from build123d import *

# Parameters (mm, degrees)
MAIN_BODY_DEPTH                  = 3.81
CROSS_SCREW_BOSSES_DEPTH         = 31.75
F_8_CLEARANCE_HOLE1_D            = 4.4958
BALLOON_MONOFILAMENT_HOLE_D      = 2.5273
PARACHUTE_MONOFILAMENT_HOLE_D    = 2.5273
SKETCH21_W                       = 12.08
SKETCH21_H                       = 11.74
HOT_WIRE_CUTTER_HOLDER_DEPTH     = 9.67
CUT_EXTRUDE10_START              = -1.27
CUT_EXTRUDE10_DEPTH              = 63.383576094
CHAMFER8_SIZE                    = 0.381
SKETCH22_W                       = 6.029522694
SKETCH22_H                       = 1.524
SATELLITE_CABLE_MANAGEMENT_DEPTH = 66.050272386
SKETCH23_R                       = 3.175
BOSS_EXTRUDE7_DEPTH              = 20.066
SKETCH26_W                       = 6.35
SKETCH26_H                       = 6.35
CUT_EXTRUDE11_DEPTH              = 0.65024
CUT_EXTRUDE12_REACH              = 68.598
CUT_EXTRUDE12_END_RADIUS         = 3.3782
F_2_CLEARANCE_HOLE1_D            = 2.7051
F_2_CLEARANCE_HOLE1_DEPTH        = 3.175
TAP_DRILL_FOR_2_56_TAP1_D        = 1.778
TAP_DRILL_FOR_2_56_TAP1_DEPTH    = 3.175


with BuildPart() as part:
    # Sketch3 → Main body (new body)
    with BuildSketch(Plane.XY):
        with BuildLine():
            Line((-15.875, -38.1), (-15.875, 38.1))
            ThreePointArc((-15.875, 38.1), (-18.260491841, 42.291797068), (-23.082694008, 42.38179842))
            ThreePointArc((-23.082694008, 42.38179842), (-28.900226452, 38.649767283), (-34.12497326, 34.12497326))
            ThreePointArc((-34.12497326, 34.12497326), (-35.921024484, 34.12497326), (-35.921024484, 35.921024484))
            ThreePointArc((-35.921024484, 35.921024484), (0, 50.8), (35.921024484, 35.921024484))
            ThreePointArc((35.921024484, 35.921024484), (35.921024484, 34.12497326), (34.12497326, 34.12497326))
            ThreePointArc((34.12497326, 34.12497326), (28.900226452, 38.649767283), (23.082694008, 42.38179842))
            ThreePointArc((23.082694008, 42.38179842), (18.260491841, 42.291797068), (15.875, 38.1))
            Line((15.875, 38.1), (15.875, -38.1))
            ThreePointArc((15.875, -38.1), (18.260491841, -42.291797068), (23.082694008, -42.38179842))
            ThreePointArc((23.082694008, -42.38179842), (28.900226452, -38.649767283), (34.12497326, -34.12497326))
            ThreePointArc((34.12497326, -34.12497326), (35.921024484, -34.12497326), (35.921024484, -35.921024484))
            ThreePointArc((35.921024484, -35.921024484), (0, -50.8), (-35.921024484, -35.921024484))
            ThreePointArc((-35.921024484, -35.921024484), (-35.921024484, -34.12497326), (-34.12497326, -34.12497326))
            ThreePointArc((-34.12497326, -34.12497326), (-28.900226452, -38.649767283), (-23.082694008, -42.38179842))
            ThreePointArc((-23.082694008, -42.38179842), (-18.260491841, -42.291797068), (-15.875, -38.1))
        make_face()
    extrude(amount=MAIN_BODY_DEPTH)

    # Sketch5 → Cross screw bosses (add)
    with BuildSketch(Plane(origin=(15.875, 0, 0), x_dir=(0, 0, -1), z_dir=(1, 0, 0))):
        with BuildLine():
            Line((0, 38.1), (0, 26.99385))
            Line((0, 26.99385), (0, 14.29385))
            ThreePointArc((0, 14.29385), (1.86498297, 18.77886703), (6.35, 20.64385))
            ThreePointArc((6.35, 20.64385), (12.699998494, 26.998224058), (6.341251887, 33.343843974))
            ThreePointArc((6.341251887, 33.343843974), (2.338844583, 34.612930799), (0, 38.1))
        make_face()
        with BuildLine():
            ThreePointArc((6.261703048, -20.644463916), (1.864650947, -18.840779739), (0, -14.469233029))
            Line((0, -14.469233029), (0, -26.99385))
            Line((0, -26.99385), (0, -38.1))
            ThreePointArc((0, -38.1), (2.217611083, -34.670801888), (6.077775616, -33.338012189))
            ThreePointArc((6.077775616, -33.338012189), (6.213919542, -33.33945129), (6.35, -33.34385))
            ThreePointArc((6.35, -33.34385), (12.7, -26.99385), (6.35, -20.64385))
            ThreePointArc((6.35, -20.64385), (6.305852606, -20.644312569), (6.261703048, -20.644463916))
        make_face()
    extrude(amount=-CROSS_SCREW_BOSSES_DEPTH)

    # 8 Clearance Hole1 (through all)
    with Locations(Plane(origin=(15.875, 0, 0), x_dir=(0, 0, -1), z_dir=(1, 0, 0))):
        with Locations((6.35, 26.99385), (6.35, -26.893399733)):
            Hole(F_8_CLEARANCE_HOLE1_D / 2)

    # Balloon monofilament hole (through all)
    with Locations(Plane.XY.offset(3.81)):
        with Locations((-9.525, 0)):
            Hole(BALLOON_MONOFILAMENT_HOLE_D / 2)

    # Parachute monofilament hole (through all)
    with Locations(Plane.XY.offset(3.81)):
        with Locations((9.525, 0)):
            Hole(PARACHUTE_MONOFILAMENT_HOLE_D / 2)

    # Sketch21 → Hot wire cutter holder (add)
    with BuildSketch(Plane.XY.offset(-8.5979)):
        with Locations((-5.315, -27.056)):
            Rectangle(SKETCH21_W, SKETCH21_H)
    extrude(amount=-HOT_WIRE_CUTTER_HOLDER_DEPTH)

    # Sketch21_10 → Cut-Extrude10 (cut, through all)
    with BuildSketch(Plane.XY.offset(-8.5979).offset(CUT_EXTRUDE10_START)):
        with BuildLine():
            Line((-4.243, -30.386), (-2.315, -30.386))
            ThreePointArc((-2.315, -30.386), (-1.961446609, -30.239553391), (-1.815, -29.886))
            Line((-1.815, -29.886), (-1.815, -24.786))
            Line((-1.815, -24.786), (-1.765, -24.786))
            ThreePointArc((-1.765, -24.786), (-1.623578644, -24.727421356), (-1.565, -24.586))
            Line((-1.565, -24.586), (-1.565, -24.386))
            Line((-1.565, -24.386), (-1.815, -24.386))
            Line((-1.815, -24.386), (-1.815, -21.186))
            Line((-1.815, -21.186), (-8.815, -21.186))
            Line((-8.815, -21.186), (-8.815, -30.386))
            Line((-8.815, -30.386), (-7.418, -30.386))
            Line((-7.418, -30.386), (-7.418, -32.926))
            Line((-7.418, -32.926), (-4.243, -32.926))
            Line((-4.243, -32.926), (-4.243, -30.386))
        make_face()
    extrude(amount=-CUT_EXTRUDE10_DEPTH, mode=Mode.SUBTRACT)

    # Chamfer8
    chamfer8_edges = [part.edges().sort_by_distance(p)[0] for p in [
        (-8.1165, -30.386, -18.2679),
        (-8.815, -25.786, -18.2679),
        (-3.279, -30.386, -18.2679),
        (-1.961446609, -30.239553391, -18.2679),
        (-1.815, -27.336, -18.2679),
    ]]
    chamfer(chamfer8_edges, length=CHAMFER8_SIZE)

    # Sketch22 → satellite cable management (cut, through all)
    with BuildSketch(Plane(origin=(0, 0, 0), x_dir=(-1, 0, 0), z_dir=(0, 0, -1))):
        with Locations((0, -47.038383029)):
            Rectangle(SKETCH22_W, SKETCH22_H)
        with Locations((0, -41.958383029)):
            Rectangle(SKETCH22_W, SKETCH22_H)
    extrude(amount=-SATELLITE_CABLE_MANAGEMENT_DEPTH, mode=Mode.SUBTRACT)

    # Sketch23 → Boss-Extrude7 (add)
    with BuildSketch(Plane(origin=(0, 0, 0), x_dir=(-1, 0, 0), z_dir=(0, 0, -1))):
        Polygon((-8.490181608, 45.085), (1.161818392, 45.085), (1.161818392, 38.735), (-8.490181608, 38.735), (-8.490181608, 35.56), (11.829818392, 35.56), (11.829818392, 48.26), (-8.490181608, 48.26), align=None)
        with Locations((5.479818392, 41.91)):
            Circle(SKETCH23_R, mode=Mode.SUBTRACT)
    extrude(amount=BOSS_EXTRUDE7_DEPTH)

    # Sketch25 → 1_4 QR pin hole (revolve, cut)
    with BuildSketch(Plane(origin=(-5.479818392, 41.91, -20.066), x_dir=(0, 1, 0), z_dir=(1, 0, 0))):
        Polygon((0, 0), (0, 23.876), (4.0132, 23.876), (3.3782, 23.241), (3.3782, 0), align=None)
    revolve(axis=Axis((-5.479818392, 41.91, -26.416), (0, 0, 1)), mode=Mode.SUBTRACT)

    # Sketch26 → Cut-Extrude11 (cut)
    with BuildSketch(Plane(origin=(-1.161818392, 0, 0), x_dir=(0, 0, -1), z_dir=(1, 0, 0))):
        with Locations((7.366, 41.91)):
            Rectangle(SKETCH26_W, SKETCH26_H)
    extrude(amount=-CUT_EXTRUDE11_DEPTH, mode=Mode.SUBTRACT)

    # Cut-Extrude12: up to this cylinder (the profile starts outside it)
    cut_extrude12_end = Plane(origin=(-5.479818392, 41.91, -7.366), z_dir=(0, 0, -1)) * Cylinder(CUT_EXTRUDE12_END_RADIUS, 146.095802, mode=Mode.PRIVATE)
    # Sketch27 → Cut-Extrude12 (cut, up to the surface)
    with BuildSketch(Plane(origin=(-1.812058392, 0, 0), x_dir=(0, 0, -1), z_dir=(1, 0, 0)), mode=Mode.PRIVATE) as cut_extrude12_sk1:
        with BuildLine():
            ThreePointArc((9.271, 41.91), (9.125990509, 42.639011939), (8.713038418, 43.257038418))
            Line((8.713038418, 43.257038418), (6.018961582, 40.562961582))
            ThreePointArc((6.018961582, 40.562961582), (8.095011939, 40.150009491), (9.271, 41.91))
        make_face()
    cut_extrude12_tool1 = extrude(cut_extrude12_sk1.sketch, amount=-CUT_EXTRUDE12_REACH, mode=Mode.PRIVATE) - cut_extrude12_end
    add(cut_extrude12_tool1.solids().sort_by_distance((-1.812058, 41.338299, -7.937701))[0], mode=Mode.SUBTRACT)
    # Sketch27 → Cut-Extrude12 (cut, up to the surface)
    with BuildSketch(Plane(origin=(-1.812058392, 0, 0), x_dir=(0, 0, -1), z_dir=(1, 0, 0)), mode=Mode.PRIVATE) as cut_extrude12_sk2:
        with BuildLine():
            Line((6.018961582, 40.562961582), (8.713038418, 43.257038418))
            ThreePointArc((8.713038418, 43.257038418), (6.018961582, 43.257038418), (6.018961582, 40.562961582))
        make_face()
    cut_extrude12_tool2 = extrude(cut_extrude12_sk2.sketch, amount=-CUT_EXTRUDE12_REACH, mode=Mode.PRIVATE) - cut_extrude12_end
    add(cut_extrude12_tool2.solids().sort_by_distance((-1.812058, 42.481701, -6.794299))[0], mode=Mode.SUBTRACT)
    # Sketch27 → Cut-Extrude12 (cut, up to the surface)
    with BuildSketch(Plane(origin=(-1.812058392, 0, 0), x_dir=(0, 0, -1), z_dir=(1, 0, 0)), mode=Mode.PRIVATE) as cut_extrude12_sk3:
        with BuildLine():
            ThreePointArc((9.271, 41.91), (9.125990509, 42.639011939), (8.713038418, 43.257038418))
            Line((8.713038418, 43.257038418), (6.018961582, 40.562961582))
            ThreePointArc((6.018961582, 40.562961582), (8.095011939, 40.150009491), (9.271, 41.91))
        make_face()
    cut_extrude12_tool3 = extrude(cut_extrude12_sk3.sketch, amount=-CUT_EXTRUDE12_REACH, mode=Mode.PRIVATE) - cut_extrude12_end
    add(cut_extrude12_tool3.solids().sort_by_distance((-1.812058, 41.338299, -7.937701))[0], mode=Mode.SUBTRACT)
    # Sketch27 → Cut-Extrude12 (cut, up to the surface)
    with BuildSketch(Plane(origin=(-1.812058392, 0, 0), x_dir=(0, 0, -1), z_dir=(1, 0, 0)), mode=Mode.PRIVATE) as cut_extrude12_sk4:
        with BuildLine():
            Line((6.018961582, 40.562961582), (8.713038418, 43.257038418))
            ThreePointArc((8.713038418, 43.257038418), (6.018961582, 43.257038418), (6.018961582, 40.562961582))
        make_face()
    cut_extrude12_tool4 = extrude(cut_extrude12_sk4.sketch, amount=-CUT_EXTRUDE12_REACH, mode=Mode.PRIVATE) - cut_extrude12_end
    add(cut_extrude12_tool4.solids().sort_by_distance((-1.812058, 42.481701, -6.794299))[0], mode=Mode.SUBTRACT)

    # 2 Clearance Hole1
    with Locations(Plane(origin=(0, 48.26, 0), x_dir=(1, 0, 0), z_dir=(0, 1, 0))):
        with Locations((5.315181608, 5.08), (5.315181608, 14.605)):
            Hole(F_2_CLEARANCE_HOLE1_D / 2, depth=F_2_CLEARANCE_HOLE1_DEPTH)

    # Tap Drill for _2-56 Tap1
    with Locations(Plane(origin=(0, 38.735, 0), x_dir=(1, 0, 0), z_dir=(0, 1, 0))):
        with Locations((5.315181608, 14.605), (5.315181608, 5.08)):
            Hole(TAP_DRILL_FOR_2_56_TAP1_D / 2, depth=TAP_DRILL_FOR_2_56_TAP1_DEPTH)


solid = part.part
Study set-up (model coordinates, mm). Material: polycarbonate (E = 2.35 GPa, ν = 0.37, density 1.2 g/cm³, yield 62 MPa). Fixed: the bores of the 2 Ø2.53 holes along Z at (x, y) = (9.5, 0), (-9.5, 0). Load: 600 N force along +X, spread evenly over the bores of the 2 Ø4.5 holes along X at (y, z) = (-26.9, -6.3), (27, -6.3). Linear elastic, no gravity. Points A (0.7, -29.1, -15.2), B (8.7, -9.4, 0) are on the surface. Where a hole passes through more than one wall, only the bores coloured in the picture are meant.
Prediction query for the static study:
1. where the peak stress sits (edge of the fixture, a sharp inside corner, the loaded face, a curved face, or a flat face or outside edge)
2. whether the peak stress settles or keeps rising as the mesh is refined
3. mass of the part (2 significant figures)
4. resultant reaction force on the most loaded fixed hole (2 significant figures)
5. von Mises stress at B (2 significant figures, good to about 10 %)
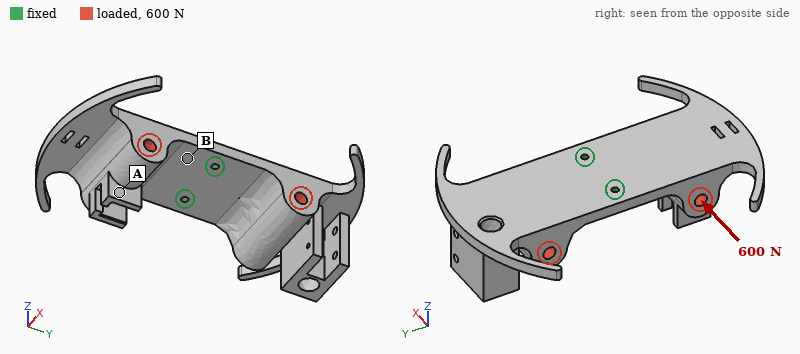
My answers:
edge of the fixture
keeps rising
31 g
380 N
18 MPa
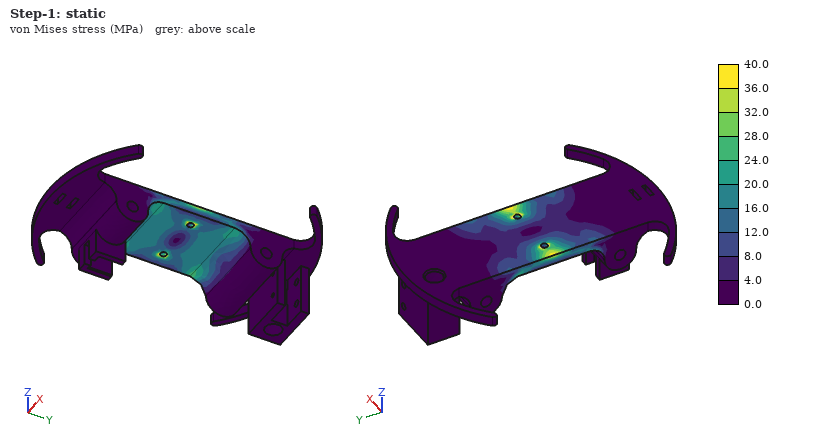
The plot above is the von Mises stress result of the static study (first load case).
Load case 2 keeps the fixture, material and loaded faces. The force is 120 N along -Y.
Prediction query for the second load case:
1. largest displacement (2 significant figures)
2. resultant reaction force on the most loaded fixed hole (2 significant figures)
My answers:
1.3 mm
60 N
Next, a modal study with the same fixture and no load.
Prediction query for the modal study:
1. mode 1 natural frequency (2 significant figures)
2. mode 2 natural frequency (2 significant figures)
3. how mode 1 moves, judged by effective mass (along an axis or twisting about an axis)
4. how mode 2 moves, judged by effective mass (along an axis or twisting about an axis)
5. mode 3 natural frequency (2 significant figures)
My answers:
200 Hz
270 Hz
along Z
along Z
730 Hz
